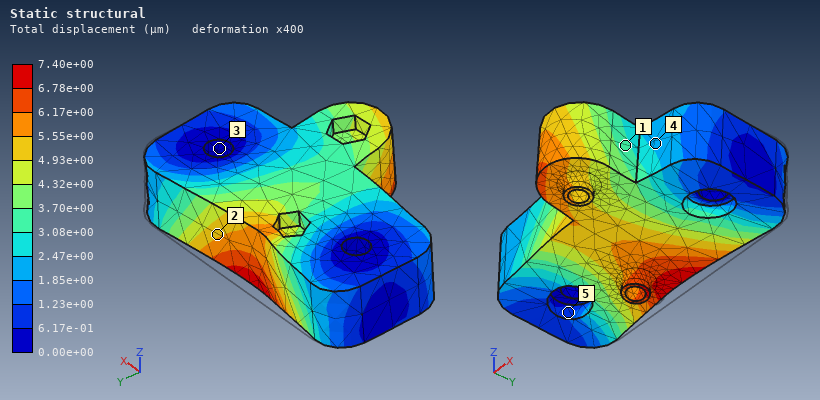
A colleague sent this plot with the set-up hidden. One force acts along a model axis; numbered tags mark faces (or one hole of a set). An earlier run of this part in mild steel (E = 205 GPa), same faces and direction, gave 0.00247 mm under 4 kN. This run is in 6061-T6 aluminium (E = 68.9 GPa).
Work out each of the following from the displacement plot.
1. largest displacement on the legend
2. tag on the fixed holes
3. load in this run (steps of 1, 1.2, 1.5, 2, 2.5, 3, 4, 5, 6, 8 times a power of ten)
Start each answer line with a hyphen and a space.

- 7.40e+00 µm
- 3
- 4 kN
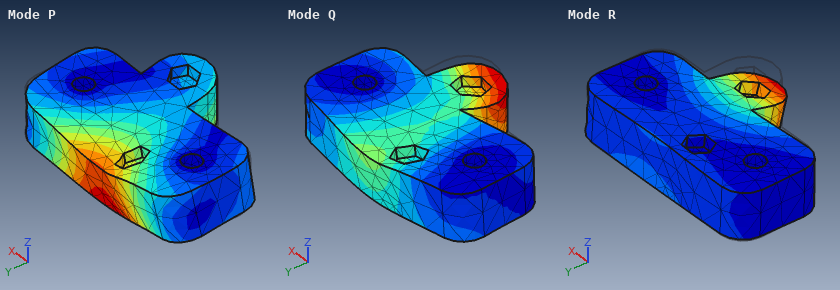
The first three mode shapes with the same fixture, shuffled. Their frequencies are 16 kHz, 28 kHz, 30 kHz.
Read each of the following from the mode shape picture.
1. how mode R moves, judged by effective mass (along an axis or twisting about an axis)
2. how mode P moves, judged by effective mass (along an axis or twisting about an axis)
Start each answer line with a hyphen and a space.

- along Z
- along Z
